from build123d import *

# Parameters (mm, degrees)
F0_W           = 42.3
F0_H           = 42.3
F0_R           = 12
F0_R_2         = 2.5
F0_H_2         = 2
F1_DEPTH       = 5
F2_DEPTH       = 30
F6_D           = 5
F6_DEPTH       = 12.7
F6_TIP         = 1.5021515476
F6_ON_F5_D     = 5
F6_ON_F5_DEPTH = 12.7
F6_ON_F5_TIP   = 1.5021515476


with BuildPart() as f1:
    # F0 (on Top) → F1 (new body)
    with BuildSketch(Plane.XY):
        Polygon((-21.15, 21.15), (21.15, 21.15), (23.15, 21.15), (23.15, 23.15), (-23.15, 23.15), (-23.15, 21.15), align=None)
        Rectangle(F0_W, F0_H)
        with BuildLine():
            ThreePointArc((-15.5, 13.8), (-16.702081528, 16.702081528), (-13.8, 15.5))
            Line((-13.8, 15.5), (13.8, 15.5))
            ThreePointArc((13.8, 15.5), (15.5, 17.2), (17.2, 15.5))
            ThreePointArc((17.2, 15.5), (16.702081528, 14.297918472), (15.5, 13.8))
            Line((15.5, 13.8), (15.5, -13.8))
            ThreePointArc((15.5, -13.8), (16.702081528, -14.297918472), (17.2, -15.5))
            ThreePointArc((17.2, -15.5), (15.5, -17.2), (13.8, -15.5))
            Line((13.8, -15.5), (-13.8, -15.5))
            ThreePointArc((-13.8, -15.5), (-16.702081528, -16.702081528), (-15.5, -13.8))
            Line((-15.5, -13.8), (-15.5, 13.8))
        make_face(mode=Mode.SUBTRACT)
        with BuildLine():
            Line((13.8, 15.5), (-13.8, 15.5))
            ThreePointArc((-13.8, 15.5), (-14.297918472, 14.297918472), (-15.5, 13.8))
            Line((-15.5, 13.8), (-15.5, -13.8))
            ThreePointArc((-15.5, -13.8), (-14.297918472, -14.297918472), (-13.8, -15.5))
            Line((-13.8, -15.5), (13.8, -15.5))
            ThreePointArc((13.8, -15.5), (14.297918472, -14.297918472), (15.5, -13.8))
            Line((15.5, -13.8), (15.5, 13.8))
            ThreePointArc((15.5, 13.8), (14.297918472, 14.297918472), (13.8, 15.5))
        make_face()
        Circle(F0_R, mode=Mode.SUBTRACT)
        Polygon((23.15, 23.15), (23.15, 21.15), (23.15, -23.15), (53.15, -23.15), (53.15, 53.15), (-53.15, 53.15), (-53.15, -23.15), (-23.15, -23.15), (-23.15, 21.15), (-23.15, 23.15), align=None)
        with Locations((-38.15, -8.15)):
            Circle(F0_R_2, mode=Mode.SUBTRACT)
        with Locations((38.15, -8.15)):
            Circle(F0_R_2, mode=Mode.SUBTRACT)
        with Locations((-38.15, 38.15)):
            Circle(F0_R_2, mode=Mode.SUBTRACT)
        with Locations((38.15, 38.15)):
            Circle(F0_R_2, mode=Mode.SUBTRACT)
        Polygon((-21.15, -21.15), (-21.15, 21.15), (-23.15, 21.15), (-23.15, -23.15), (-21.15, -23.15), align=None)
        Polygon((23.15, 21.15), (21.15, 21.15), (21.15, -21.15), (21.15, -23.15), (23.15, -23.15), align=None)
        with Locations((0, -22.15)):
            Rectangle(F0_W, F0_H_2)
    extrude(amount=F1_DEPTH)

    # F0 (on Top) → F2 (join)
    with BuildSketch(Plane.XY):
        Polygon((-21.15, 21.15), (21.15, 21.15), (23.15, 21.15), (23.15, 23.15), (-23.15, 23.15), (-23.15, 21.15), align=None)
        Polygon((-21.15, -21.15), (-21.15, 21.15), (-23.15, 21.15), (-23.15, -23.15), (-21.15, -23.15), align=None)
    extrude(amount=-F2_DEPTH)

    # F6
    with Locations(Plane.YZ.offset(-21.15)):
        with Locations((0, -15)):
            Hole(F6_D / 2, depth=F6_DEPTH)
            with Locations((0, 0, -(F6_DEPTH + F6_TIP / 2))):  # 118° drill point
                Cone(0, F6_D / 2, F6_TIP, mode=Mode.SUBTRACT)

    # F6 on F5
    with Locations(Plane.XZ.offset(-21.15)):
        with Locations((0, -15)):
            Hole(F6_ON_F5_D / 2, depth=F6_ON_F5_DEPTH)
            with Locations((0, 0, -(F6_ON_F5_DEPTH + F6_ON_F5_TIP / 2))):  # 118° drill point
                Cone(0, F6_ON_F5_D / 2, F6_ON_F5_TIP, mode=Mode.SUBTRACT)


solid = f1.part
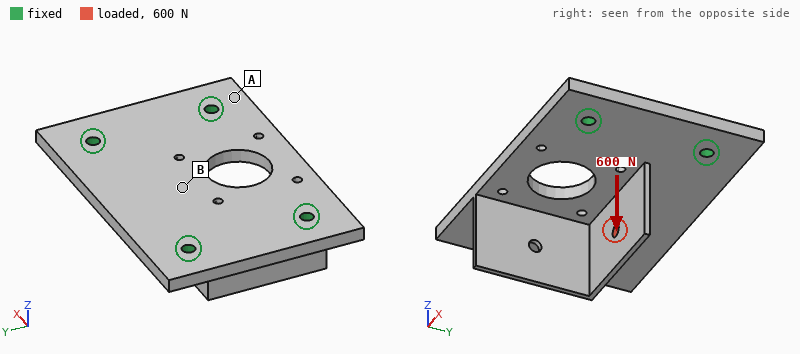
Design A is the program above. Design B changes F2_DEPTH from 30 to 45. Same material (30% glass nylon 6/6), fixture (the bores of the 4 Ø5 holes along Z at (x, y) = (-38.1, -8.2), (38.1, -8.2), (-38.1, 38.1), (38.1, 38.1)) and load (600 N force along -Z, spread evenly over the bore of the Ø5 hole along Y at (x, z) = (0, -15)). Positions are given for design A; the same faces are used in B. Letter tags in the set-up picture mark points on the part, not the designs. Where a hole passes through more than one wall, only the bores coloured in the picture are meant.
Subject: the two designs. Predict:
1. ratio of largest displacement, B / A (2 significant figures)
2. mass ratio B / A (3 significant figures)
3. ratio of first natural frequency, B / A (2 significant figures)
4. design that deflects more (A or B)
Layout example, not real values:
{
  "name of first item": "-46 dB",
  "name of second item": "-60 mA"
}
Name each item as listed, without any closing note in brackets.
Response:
{
  "ratio of largest displacement, B / A": "1.1",
  "mass ratio B / A": "1.06",
  "ratio of first natural frequency, B / A": "0.55",
  "design that deflects more": "B"
}
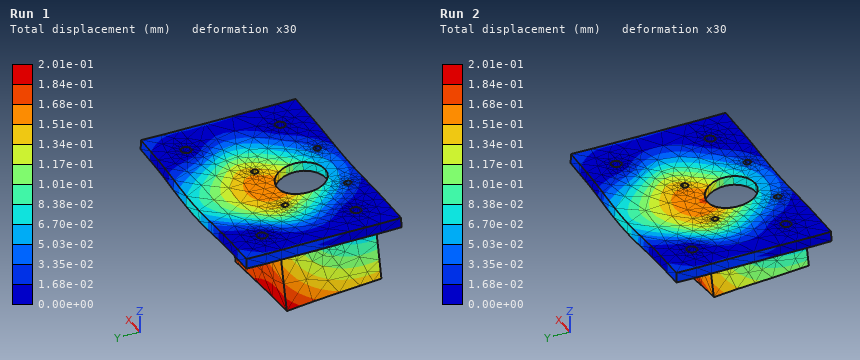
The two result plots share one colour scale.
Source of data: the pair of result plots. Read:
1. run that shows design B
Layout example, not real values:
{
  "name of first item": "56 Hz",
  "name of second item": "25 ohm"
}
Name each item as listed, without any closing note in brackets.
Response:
{
  "run that shows design B": "Run 1"
}
